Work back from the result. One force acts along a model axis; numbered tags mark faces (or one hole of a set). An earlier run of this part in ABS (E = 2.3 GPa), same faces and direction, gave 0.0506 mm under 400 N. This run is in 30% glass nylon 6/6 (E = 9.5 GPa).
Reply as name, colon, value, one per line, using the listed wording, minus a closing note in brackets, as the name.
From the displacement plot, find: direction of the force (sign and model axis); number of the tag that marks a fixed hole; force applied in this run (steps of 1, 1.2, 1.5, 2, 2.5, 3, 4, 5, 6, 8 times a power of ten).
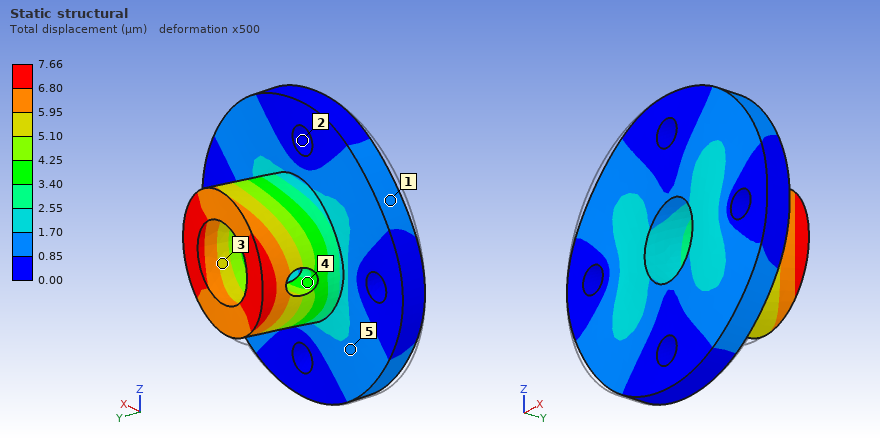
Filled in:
direction of the force: +X
number of the tag that marks a fixed hole: 2
force applied in this run: 250 N
